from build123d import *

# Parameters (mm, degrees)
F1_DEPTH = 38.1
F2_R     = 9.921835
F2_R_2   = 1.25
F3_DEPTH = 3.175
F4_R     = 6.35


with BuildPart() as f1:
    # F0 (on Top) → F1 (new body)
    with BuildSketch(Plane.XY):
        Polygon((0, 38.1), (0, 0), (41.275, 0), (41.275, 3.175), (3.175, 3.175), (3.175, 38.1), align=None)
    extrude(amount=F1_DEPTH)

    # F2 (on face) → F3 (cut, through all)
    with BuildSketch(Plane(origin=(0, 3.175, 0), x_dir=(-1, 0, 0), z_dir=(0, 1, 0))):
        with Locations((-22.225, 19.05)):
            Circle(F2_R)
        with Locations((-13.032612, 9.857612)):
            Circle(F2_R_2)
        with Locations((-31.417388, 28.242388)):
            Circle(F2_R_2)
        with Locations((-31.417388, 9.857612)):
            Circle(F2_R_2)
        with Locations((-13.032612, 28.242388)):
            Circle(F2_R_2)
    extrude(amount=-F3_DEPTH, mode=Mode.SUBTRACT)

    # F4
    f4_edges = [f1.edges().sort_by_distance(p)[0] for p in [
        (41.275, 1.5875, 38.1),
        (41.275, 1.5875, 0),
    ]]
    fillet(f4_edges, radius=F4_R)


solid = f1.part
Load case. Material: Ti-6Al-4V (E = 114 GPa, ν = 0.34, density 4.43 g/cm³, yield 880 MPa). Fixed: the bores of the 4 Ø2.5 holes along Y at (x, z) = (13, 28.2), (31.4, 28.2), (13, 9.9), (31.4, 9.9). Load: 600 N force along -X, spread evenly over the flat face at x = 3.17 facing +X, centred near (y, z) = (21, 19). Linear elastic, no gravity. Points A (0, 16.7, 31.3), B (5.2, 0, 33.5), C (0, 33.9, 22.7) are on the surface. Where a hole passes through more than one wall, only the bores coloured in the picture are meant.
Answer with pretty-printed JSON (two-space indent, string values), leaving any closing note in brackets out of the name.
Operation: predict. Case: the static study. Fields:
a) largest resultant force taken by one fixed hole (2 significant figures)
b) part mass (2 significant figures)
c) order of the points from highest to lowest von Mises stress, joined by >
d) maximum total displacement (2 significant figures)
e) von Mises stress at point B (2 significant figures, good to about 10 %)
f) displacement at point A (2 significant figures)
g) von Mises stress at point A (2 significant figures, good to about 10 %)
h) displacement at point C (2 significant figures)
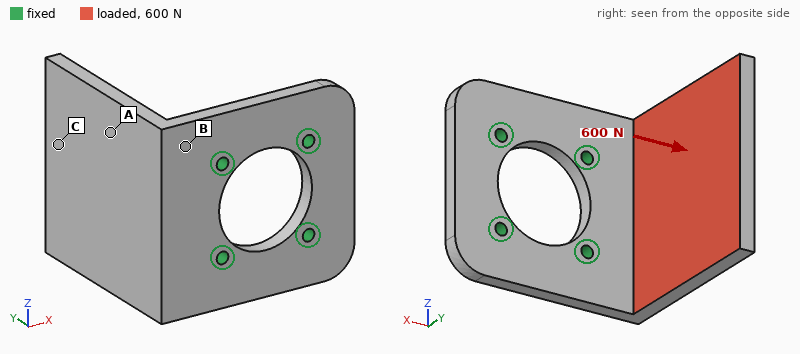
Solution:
{
  "largest resultant force taken by one fixed hole": "320 N",
  "part mass": "36 g",
  "order of the points from highest to lowest von Mises stress, joined by >": "B > A > C",
  "maximum total displacement": "0.73 mm",
  "von Mises stress at point B": "150 MPa",
  "displacement at point A": "0.27 mm",
  "von Mises stress at point A": "59 MPa",
  "displacement at point C": "0.64 mm"
}
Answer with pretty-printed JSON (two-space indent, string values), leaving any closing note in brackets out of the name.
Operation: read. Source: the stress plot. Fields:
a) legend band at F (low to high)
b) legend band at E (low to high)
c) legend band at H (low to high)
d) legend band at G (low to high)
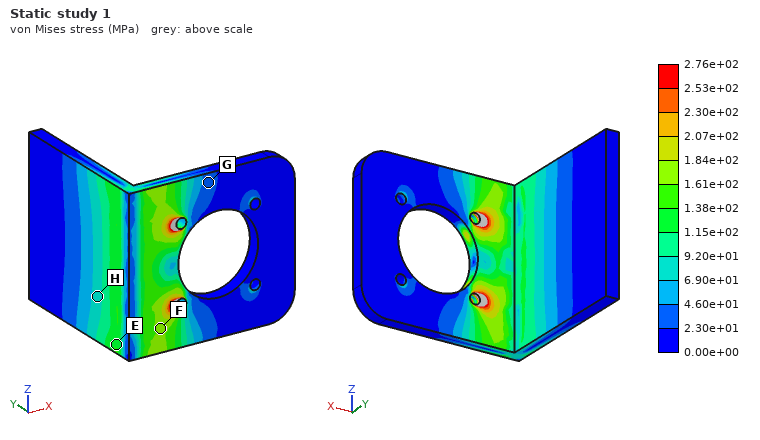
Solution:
{
  "legend band at F": "1.61e+02 to 1.84e+02 MPa",
  "legend band at E": "1.15e+02 to 1.38e+02 MPa",
  "legend band at H": "6.90e+01 to 9.20e+01 MPa",
  "legend band at G": "2.30e+01 to 4.60e+01 MPa"
}
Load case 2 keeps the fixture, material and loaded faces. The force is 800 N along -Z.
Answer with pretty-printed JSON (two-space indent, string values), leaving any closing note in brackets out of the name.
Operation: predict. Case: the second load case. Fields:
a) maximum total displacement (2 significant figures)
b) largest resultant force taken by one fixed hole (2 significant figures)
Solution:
{
  "maximum total displacement": "0.17 mm",
  "largest resultant force taken by one fixed hole": "860 N"
}
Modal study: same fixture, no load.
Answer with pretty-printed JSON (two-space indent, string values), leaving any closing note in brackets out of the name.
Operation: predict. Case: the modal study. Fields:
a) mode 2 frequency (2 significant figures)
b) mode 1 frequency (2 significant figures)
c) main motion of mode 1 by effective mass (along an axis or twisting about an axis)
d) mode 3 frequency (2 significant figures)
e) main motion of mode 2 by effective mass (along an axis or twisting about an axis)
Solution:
{
  "mode 2 frequency": "2900 Hz",
  "mode 1 frequency": "1300 Hz",
  "main motion of mode 1 by effective mass": "along X",
  "mode 3 frequency": "4500 Hz",
  "main motion of mode 2 by effective mass": "along Z"
}
